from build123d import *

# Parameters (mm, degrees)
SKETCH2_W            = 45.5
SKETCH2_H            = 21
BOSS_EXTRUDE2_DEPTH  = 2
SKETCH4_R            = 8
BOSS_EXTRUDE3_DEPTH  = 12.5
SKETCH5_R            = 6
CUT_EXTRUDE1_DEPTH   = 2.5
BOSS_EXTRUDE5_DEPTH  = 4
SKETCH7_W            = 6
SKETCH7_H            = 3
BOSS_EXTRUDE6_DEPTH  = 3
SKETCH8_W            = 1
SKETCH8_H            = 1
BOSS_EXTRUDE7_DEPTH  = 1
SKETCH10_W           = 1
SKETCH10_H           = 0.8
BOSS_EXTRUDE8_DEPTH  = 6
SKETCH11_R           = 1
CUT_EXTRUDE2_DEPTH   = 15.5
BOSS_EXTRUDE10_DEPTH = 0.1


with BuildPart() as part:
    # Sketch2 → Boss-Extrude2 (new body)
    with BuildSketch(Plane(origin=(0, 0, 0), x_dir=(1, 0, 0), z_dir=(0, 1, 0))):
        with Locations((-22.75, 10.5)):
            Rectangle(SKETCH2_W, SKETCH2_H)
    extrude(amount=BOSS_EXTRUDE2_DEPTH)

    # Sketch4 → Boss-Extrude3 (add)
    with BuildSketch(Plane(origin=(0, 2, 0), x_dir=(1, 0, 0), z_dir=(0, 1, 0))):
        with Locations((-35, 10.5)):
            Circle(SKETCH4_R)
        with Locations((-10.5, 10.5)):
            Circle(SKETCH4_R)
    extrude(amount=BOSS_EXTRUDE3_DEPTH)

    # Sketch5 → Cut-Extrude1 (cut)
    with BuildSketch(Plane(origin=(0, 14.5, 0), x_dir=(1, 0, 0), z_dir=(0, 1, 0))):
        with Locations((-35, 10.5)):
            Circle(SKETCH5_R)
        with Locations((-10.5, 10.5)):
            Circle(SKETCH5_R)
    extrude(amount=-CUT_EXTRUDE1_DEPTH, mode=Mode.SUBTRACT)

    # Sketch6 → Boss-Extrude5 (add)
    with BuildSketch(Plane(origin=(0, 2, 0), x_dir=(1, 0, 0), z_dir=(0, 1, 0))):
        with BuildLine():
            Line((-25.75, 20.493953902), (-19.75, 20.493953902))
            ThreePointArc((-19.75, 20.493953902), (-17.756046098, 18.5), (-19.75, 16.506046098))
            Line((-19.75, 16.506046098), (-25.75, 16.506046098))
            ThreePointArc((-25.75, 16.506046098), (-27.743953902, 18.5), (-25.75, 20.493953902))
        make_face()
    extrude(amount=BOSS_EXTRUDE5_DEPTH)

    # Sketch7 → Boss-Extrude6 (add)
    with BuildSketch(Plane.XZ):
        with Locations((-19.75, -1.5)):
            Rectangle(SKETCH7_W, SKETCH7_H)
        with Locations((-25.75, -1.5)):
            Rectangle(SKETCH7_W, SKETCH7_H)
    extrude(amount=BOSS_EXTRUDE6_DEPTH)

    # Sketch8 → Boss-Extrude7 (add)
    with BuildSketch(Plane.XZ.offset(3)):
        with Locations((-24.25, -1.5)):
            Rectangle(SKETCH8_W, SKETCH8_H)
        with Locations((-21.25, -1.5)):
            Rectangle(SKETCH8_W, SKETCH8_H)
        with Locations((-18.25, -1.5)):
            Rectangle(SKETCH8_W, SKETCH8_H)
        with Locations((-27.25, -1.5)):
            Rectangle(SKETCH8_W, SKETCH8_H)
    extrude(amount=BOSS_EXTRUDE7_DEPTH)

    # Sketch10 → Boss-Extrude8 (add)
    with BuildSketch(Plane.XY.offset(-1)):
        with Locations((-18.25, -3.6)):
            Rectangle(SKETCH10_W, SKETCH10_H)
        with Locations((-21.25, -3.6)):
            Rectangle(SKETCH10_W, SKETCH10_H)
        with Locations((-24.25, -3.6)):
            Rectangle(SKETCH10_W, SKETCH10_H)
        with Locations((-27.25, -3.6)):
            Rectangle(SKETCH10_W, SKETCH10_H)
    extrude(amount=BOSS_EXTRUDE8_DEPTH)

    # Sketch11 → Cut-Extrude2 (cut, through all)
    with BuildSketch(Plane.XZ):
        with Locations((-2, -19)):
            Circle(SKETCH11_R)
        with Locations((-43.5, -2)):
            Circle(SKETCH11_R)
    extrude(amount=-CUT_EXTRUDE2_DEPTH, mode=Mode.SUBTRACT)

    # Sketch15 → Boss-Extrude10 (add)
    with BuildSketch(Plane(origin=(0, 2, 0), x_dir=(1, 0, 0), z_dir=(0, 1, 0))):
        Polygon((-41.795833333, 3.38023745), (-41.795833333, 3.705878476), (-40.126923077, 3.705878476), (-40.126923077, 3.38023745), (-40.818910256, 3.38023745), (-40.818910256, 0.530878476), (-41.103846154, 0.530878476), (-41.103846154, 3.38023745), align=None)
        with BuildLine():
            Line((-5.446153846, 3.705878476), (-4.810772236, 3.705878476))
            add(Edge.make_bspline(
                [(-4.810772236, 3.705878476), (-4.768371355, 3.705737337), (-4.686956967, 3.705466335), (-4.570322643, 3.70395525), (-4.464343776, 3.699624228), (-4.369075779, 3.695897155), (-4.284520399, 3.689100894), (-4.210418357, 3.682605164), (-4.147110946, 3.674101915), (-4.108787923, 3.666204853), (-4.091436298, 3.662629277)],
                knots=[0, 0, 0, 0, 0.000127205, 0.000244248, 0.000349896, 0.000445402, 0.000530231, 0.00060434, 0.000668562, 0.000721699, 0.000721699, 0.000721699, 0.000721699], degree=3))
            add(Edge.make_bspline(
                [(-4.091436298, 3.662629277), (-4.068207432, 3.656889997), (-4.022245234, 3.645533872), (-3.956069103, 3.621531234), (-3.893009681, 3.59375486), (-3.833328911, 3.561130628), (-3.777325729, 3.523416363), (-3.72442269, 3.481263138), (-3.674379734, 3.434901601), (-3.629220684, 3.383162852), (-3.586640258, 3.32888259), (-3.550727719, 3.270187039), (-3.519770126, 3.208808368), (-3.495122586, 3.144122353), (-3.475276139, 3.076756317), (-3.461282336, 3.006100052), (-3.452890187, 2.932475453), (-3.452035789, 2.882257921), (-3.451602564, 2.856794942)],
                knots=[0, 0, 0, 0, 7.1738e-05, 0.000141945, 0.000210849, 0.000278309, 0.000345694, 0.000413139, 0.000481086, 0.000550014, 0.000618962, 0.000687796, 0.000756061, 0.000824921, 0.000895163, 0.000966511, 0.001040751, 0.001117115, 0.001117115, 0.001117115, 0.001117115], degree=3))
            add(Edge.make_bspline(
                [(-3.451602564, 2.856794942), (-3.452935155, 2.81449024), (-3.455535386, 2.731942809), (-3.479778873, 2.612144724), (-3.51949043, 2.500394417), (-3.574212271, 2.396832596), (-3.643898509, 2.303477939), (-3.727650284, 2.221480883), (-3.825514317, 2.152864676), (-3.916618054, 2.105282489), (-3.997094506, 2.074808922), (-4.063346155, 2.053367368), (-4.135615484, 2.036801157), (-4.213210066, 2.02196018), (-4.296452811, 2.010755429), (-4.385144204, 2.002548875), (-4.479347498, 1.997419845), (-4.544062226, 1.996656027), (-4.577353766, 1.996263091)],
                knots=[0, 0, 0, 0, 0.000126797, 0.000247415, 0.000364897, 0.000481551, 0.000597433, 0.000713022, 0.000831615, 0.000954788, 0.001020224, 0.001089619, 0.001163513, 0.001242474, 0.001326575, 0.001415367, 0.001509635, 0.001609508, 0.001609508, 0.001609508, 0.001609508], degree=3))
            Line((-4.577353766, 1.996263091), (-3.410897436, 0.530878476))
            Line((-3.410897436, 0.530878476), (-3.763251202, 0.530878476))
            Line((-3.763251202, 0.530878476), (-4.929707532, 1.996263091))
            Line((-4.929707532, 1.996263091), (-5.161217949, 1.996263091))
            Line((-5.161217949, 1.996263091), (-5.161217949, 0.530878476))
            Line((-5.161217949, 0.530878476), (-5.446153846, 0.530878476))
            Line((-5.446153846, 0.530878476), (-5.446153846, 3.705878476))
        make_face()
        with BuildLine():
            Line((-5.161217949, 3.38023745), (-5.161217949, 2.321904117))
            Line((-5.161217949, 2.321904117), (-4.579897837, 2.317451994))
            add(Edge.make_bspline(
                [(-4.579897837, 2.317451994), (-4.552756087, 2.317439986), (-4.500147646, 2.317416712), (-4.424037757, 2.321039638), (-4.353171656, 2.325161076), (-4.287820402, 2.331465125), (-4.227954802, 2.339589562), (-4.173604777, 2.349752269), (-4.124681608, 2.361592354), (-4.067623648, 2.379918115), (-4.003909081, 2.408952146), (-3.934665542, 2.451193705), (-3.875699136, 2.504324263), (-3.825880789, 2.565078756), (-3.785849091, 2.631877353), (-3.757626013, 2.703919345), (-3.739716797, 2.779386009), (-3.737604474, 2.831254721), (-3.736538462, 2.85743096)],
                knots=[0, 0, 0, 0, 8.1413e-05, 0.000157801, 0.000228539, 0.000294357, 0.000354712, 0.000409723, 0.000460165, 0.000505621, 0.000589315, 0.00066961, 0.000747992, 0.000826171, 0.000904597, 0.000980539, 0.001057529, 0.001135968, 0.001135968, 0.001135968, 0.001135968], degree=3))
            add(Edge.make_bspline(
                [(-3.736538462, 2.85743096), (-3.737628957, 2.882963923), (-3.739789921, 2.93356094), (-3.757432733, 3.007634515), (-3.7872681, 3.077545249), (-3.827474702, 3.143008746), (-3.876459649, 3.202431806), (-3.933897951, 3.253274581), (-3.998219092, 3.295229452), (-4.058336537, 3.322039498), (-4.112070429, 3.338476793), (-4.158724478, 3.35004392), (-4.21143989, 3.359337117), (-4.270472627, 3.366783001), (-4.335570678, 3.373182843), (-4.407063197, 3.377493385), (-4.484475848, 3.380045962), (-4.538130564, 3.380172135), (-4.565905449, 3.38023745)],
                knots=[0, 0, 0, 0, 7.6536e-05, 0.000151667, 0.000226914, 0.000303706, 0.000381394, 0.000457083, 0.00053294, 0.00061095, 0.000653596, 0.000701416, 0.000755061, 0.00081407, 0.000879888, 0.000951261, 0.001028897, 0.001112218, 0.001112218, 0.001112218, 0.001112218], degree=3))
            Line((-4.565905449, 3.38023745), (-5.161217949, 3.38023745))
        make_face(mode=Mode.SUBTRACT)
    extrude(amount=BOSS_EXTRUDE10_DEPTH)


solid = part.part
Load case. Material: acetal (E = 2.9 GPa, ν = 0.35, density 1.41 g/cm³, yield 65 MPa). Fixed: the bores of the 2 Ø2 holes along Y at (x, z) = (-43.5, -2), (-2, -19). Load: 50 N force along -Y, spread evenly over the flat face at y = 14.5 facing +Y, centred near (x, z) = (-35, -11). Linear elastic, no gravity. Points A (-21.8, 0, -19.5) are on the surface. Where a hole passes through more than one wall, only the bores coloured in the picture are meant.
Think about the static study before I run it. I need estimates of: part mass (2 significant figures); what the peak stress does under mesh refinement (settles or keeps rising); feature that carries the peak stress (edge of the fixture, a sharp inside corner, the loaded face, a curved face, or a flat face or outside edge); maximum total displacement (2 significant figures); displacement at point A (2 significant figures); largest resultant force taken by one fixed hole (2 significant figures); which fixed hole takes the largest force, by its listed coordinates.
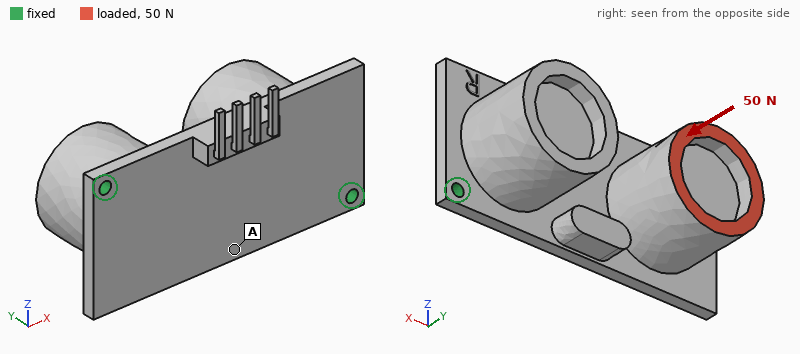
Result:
9.4 g
keeps rising
edge of the fixture
0.59 mm
0.38 mm
39 N
(-43.5, -2)
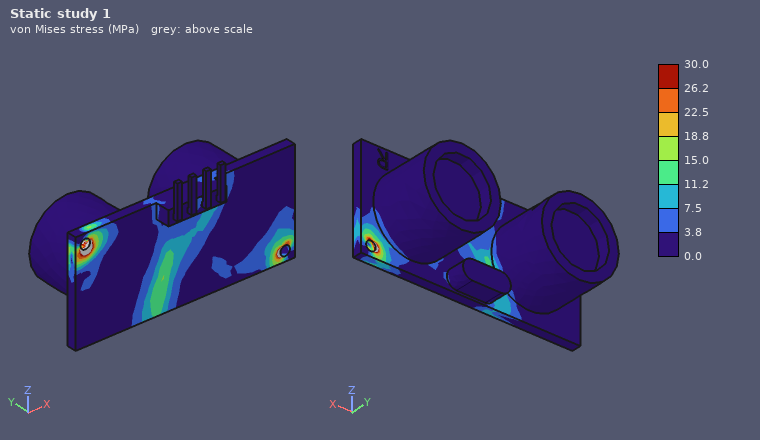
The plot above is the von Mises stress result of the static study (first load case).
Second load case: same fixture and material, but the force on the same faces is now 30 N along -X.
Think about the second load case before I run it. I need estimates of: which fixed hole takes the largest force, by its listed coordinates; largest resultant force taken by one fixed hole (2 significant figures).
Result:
(-43.5, -2)
19 N
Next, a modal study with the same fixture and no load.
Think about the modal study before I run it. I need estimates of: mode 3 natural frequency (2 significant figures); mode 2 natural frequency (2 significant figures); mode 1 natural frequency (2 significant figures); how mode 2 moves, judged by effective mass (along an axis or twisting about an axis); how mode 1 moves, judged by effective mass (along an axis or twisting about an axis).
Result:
1400 Hz
750 Hz
600 Hz
along Y
along Z
